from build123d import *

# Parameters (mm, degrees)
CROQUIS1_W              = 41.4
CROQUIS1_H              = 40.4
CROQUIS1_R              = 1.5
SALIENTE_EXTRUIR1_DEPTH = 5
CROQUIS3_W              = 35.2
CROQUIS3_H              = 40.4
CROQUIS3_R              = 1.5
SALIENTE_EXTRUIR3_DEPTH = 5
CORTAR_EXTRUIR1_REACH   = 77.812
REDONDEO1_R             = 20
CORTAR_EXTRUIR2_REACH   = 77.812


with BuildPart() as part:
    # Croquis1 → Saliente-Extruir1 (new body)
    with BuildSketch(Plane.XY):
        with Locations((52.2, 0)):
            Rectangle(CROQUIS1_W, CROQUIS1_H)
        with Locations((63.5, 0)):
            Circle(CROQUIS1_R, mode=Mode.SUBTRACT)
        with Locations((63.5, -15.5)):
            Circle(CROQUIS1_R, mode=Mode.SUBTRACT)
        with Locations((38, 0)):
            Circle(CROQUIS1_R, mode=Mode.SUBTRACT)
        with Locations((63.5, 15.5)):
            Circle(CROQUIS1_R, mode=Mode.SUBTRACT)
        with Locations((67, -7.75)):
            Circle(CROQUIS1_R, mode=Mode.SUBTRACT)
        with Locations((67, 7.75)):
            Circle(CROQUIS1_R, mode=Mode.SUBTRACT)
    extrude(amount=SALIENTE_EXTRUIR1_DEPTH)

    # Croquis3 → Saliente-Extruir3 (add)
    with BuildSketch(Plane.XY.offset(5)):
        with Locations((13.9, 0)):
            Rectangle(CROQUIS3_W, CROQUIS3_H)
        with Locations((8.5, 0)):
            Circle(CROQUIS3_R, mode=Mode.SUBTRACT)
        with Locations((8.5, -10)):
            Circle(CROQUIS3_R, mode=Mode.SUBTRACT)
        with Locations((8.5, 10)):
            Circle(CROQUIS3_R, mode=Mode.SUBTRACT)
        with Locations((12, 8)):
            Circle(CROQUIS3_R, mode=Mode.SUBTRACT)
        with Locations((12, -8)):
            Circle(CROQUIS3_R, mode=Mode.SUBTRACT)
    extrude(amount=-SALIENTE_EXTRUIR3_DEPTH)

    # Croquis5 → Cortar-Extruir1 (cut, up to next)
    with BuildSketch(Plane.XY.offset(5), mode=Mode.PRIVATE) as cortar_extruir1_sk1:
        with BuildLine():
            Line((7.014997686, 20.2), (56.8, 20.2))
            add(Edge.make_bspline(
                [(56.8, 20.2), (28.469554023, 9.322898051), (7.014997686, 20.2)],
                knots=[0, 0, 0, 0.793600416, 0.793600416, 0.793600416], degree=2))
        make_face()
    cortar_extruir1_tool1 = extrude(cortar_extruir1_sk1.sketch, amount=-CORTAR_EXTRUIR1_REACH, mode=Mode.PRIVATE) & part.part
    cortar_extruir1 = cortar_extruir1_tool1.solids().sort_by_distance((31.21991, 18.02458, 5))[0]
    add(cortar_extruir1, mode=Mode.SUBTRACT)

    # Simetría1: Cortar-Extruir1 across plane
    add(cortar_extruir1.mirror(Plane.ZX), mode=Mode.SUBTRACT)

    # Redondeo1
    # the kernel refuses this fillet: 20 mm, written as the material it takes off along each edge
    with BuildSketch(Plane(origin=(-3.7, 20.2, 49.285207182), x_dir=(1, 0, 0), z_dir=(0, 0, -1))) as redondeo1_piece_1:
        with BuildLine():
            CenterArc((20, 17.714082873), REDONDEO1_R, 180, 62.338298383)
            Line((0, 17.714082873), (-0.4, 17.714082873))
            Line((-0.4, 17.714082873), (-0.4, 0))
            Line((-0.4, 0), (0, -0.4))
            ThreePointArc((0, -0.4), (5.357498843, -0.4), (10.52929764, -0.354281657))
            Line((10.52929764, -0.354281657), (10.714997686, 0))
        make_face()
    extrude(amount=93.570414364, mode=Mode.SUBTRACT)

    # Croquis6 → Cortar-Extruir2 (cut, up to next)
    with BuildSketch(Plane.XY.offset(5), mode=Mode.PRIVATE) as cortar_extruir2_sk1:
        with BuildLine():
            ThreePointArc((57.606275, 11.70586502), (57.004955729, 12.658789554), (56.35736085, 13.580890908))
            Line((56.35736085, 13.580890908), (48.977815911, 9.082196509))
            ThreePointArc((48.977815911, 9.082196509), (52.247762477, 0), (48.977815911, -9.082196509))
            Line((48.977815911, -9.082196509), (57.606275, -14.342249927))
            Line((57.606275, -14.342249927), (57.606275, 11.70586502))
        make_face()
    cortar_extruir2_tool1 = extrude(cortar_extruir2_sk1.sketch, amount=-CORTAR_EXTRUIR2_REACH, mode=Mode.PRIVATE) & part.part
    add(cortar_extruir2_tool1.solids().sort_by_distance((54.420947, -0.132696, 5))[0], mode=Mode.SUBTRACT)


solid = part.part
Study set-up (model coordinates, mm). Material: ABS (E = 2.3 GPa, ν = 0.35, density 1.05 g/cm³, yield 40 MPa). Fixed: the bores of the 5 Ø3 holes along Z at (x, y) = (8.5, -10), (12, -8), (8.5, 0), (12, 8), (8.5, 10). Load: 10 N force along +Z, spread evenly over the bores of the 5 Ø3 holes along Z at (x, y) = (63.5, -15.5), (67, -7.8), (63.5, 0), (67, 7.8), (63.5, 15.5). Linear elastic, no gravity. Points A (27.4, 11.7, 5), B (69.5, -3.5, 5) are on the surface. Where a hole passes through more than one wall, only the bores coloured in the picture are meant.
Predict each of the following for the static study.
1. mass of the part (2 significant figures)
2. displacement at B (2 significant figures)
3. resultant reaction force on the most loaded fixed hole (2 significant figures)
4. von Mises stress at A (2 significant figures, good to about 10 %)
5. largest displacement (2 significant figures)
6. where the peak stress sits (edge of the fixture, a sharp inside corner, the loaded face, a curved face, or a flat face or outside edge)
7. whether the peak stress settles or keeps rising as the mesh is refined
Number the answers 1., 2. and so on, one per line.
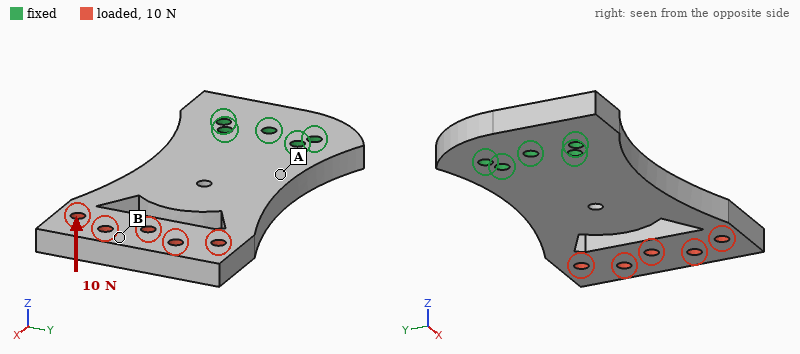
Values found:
1. 13 g
2. 0.81 mm
3. 20 N
4. 3.1 MPa
5. 0.89 mm
6. edge of the fixture
7. keeps rising
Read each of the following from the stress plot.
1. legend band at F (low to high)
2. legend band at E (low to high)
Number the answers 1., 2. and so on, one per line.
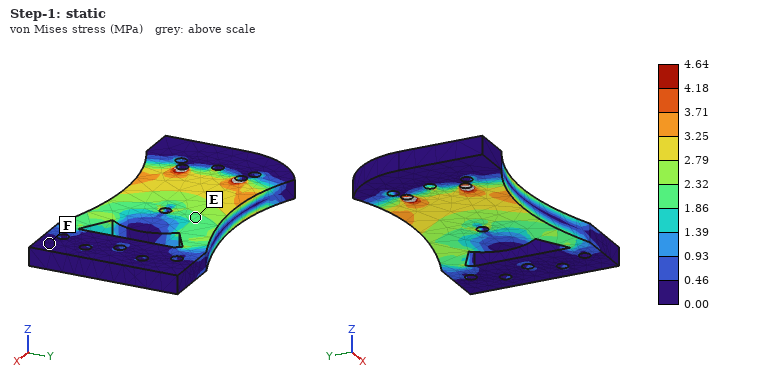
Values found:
1. 0.00 to 0.46 MPa
2. 1.86 to 2.32 MPa
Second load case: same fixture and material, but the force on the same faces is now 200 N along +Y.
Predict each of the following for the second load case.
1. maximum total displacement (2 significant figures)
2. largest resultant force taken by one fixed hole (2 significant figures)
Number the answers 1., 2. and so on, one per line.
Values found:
1. 0.86 mm
2. 320 N
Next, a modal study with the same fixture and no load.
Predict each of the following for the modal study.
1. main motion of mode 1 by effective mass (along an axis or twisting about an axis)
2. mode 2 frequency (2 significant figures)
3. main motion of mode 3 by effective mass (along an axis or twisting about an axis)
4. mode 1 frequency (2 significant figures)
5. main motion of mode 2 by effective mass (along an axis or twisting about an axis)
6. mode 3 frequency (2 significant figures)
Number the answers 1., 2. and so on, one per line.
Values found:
1. along Z
2. 920 Hz
3. along Y
4. 300 Hz
5. twisting about X
6. 1300 Hz
